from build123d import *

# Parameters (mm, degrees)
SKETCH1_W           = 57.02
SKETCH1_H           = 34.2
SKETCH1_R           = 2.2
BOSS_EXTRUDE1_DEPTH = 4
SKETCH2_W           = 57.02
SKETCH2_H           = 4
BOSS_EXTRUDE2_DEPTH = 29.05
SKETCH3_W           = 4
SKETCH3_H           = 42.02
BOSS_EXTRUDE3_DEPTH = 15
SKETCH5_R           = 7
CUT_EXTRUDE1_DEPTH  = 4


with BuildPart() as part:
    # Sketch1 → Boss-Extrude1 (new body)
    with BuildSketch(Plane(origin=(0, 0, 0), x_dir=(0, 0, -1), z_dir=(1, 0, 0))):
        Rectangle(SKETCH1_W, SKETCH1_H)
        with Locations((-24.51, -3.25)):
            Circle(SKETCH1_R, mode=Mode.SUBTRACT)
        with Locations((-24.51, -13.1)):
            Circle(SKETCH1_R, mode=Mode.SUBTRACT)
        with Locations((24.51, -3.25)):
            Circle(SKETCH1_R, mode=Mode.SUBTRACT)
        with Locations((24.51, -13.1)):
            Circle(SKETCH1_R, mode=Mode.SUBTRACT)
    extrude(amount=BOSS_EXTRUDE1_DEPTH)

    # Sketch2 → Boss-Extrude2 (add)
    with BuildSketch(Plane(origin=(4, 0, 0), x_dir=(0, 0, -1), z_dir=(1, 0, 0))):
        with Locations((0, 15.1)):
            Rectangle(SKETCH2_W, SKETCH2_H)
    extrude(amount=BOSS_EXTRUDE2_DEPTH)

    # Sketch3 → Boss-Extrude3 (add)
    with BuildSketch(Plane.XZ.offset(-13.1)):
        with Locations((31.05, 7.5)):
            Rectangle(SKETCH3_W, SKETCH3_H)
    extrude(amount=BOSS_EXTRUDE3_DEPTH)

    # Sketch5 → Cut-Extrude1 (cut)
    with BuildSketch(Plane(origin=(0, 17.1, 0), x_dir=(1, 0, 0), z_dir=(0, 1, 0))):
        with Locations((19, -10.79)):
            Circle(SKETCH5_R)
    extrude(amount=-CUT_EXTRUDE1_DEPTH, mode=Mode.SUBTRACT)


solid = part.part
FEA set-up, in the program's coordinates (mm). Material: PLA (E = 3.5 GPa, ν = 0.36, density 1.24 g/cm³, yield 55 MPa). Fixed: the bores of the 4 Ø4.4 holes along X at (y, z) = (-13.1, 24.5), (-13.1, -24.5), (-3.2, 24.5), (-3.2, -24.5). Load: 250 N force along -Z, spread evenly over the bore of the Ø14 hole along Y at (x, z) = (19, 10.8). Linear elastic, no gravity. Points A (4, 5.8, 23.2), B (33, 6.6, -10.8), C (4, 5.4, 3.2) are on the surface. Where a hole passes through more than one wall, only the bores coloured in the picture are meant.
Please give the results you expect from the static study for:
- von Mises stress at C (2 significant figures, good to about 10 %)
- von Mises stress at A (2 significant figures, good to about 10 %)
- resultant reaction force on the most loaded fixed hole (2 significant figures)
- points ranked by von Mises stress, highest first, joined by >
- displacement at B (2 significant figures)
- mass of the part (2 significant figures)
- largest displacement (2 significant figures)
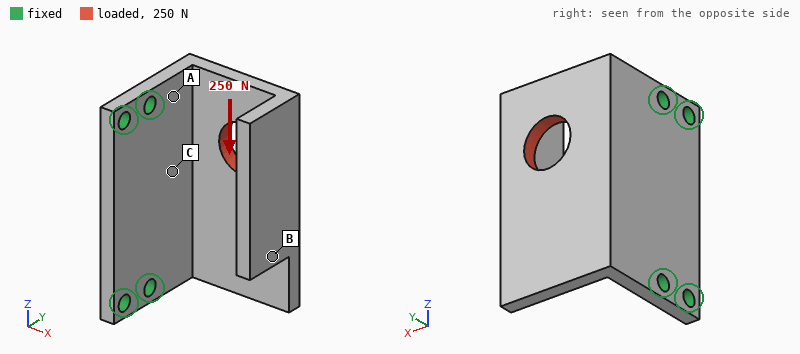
7.4 MPa
11 MPa
170 N
A > C > B
0.51 mm
20 g
0.69 mm
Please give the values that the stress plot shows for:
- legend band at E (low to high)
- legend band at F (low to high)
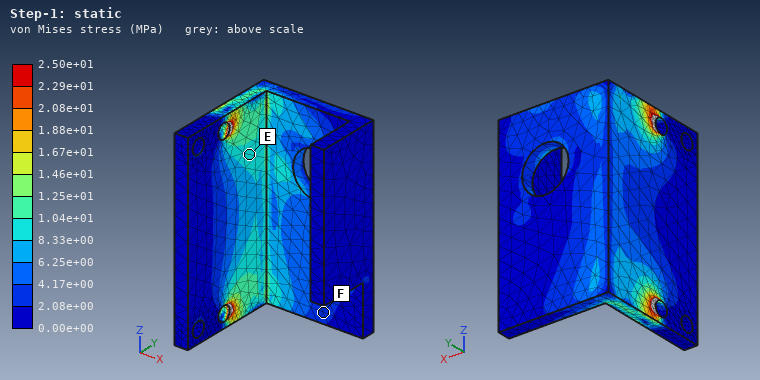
8.33e+00 to 1.04e+01 MPa
2.08e+00 to 4.17e+00 MPa
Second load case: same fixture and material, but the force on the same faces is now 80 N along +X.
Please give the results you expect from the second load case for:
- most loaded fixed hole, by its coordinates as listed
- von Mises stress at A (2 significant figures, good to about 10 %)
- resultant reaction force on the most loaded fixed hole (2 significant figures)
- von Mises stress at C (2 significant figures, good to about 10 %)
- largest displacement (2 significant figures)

(-3.2, 24.5)
7.8 MPa
84 N
3.5 MPa
0.59 mm
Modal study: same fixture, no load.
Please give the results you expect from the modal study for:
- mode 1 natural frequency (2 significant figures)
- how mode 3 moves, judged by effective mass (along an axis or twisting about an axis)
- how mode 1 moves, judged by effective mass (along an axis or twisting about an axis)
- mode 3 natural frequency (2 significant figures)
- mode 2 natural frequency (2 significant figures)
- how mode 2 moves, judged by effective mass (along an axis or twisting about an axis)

410 Hz
along X
along Y
1100 Hz
790 Hz
along Z
